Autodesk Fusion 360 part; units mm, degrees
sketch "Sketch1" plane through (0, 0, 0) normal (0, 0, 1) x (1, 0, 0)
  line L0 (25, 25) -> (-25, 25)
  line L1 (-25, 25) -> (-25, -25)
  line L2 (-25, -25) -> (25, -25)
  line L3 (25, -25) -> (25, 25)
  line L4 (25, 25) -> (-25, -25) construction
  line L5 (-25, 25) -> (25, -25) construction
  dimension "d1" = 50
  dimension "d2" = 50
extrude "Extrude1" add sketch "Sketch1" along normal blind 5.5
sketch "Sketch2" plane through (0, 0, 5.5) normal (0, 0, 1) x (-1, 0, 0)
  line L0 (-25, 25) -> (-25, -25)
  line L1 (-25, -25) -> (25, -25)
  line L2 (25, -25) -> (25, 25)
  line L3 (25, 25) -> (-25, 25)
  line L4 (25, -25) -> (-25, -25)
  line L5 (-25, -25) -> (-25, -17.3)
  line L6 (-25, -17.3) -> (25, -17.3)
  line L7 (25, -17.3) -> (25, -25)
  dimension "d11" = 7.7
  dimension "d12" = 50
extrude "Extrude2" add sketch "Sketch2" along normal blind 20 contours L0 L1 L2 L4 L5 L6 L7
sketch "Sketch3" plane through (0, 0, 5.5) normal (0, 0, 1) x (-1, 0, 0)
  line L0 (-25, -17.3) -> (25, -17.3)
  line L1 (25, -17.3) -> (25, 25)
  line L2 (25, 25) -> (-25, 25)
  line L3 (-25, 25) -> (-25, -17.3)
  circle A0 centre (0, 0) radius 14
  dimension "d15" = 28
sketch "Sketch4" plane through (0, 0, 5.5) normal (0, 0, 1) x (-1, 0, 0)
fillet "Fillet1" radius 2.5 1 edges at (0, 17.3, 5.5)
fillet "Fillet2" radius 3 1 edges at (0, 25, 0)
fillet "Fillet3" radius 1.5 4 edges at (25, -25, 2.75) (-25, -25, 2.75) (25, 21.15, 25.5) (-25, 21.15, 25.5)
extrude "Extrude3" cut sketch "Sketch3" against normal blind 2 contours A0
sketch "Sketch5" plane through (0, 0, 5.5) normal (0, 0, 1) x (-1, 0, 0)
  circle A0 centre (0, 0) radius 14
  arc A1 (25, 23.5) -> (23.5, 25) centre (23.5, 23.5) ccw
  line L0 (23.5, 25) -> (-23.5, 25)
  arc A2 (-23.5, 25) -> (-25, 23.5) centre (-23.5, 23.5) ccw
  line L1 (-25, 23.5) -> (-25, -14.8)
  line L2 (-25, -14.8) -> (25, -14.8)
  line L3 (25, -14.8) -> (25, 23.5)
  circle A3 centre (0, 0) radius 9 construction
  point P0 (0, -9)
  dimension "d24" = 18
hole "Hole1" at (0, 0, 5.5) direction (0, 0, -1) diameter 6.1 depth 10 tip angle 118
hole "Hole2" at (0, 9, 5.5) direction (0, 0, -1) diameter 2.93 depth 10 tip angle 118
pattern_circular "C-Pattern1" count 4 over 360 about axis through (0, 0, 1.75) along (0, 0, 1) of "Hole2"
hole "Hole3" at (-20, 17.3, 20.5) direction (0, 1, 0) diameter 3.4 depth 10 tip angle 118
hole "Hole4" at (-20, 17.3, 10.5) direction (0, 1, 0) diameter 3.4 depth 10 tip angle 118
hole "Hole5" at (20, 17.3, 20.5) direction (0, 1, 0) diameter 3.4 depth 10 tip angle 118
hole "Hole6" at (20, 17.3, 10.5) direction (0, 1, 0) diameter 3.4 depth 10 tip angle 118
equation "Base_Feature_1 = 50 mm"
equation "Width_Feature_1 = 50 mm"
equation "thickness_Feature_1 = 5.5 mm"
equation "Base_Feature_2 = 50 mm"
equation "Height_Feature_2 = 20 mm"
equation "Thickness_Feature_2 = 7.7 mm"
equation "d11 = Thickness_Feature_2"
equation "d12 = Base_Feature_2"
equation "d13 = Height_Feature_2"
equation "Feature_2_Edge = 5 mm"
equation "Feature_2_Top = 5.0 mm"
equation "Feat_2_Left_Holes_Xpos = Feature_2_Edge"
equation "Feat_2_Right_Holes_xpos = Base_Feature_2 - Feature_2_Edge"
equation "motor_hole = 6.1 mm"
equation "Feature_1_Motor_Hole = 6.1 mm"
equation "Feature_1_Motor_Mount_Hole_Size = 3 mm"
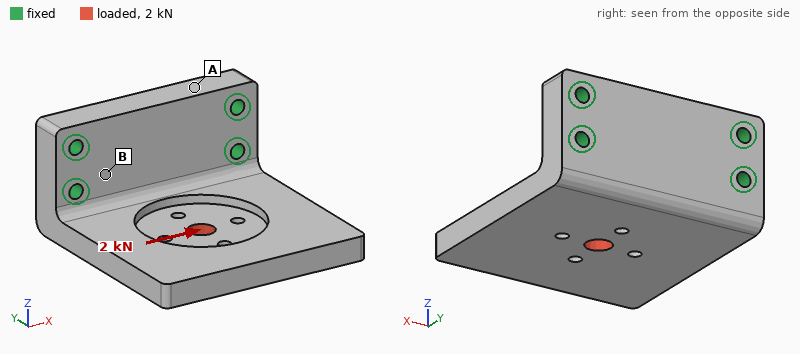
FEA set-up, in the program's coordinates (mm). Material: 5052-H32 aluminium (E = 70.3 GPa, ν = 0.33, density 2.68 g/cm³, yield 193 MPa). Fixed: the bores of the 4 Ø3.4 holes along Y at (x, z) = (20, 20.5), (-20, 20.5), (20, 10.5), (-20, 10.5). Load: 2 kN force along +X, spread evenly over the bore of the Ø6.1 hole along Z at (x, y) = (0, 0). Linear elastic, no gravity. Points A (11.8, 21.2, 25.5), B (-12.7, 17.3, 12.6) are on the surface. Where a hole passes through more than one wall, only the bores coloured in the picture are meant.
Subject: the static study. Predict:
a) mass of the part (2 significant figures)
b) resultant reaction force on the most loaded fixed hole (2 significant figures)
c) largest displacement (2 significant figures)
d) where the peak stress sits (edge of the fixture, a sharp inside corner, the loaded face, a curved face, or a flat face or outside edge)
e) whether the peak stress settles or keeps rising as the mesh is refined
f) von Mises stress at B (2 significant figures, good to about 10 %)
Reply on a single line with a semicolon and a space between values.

53 g; 1.4 kN; 32 µm; edge of the fixture; keeps rising; 12 MPa
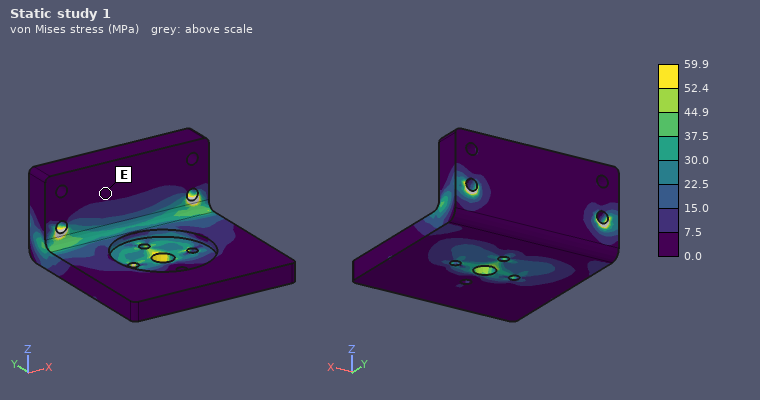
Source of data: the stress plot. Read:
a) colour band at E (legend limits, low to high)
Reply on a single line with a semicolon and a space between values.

0.0 to 7.5 MPa
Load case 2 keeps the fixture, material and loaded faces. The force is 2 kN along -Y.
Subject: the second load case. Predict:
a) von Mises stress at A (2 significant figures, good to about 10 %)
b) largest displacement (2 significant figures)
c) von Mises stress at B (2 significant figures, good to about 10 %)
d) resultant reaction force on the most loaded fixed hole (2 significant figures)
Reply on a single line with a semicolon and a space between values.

8.2 MPa; 72 µm; 18 MPa; 1.2 kN
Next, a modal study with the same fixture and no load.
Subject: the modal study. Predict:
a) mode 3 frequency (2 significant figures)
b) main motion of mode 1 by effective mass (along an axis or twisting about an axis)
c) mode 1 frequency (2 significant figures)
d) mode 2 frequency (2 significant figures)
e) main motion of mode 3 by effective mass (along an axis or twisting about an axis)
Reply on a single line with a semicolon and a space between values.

8300 Hz; along Z; 1900 Hz; 4200 Hz; along X
